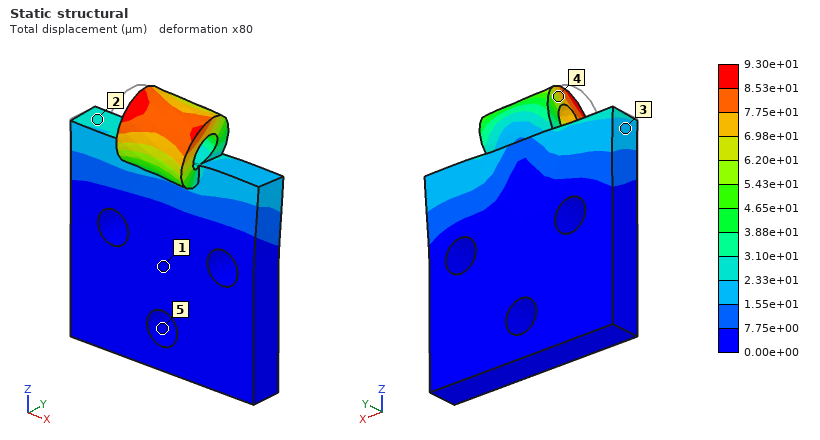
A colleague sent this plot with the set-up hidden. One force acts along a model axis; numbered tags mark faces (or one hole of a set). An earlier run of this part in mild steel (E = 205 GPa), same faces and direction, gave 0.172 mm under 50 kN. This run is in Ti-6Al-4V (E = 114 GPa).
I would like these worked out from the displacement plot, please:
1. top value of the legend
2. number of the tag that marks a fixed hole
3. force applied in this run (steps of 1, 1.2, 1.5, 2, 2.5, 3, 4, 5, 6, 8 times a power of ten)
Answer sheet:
9.30e+01 µm
5
15 kN
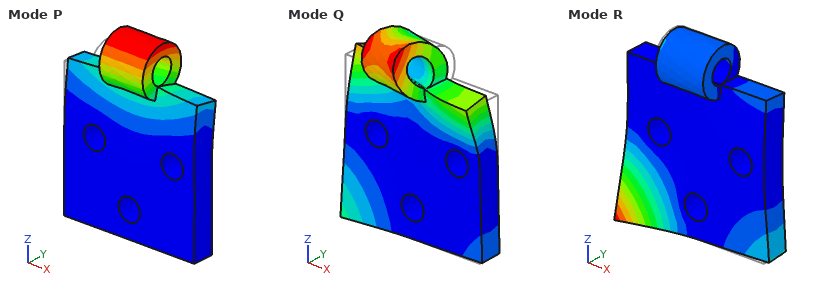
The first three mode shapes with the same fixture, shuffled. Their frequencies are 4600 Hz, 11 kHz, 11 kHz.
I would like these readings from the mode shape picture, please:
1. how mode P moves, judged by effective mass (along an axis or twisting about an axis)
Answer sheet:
along Y
